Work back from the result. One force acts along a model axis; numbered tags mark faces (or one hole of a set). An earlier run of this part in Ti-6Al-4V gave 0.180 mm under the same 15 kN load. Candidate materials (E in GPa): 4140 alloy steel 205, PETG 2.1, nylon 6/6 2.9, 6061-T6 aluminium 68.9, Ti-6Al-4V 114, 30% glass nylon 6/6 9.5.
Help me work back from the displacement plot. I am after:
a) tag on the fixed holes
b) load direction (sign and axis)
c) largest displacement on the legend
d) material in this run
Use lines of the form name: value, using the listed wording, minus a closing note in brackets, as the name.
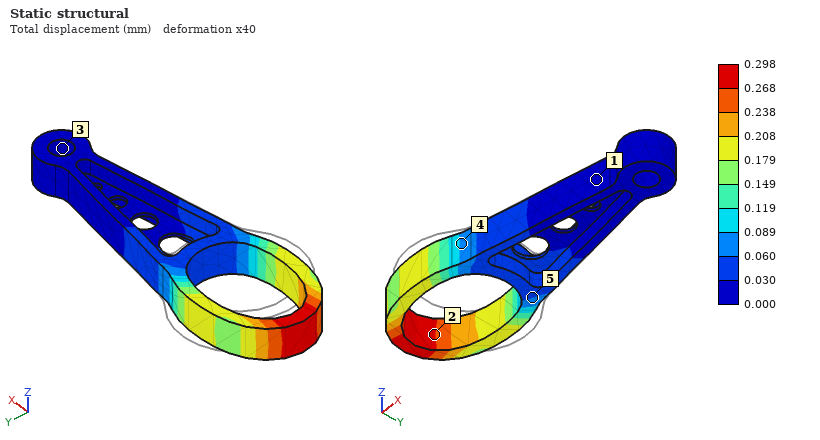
tag on the fixed holes: 3
load direction: -X
largest displacement on the legend: 0.298 mm
material in this run: 6061-T6 aluminium
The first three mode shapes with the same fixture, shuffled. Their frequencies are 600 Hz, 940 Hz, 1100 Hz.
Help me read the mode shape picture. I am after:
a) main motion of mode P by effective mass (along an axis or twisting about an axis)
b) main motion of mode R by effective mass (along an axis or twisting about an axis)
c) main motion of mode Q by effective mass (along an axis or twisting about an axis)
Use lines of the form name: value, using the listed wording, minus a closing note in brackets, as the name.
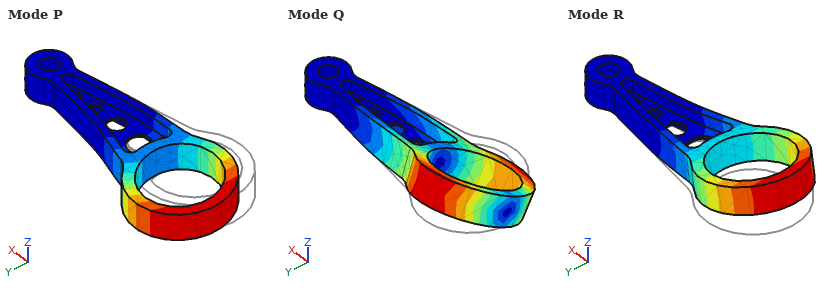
main motion of mode P by effective mass: along Y
main motion of mode R by effective mass: along Z
main motion of mode Q by effective mass: twisting about X
